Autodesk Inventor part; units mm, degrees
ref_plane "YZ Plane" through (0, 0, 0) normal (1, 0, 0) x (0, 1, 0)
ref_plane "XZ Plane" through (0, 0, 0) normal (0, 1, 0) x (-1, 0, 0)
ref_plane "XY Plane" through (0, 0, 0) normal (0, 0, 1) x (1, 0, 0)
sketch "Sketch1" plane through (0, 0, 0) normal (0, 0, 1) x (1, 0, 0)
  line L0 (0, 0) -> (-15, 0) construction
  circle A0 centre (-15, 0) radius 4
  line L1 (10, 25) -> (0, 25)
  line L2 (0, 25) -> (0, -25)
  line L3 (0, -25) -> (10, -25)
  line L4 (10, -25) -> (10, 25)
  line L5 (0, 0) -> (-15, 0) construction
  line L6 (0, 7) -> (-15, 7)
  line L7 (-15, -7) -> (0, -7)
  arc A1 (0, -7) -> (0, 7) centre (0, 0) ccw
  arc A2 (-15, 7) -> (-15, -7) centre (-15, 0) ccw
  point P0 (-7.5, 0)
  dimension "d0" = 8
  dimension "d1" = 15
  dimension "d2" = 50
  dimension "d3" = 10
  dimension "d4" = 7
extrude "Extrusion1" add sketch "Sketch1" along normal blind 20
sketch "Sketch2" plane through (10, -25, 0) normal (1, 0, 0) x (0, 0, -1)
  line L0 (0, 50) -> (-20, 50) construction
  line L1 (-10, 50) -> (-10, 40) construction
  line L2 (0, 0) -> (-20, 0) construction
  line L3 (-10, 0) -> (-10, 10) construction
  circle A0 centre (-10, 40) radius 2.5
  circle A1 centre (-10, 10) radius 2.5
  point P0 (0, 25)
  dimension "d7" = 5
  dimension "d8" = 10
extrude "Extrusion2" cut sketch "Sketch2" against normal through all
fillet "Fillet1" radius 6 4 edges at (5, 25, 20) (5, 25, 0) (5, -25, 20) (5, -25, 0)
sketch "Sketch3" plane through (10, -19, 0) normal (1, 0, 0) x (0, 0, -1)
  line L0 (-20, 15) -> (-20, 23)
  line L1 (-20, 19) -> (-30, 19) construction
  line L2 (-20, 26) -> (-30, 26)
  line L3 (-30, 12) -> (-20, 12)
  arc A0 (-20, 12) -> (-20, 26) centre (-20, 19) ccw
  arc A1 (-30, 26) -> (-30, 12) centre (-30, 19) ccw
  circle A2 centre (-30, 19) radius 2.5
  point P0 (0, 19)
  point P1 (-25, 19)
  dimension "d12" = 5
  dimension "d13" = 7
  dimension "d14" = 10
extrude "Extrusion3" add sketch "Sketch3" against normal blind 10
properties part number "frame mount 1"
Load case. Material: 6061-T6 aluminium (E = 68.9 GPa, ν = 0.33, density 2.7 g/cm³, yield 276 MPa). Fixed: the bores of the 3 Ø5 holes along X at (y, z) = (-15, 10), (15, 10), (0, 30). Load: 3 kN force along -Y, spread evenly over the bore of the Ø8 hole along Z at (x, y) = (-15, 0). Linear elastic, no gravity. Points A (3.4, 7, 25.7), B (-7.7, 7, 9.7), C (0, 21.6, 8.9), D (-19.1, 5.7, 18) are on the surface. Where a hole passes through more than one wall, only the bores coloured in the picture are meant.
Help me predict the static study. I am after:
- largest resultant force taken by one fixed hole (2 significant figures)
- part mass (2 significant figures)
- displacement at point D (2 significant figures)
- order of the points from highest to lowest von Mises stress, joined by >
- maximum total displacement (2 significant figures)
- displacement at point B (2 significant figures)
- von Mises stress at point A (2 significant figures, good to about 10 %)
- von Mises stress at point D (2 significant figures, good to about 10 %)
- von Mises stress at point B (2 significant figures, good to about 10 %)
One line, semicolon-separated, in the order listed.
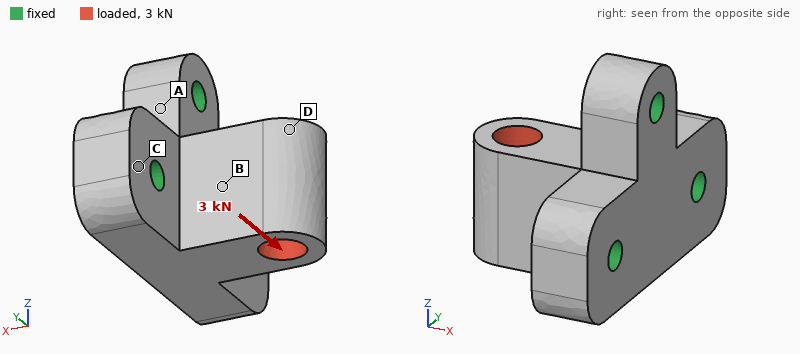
2.7 kN; 43 g; 56 µm; B > D > A > C; 60 µm; 22 µm; 17 MPa; 31 MPa; 45 MPa
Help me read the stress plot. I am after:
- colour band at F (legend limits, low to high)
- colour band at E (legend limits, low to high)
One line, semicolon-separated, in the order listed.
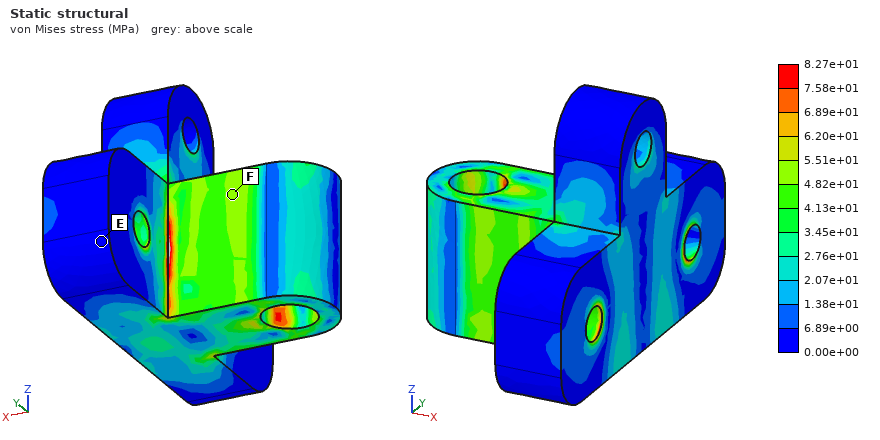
4.82e+01 to 5.51e+01 MPa; 0.00e+00 to 6.89e+00 MPa
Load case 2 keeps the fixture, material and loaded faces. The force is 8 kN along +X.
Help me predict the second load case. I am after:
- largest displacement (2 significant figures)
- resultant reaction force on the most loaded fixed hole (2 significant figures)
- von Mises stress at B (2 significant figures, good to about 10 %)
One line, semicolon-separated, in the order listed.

36 µm; 3.5 kN; 44 MPa
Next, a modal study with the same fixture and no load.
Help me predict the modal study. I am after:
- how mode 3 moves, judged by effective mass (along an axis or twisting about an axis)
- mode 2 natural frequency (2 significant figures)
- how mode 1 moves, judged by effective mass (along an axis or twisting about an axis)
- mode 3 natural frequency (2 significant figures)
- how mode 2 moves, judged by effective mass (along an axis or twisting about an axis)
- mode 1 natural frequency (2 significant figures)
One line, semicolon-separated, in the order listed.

along X; 16 kHz; along Z; 28 kHz; along Y; 15 kHz
